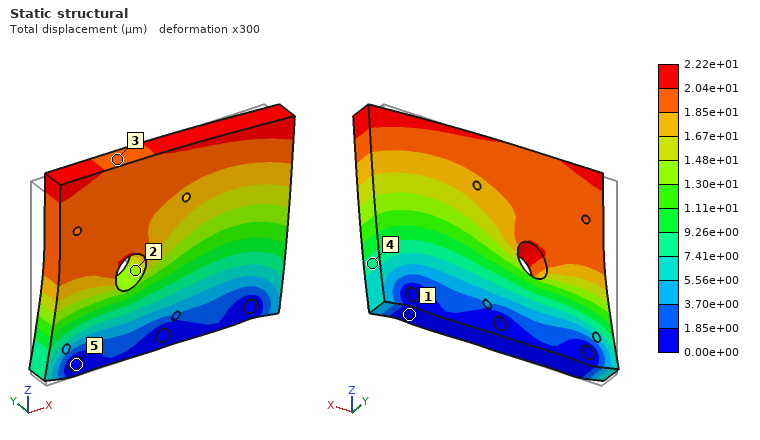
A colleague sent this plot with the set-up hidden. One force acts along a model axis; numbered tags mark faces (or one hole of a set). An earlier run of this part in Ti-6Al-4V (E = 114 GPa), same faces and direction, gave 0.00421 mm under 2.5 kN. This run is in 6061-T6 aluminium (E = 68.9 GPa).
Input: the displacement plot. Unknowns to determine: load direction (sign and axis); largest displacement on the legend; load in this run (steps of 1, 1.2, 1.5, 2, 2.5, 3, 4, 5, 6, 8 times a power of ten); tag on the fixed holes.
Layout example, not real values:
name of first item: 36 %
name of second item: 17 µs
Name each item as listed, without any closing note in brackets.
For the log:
load direction: +X
largest displacement on the legend: 2.22e+01 µm
load in this run: 8 kN
tag on the fixed holes: 5
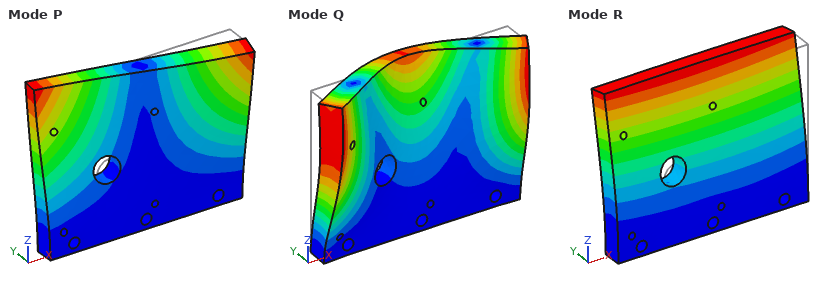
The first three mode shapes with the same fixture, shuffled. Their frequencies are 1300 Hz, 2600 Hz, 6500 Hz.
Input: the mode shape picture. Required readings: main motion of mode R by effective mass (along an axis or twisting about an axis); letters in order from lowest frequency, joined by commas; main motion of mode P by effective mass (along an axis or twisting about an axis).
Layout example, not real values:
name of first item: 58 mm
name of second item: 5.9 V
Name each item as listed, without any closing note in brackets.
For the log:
main motion of mode R by effective mass: along Y
letters in order from lowest frequency, joined by commas: R, P, Q
main motion of mode P by effective mass: twisting about Z
